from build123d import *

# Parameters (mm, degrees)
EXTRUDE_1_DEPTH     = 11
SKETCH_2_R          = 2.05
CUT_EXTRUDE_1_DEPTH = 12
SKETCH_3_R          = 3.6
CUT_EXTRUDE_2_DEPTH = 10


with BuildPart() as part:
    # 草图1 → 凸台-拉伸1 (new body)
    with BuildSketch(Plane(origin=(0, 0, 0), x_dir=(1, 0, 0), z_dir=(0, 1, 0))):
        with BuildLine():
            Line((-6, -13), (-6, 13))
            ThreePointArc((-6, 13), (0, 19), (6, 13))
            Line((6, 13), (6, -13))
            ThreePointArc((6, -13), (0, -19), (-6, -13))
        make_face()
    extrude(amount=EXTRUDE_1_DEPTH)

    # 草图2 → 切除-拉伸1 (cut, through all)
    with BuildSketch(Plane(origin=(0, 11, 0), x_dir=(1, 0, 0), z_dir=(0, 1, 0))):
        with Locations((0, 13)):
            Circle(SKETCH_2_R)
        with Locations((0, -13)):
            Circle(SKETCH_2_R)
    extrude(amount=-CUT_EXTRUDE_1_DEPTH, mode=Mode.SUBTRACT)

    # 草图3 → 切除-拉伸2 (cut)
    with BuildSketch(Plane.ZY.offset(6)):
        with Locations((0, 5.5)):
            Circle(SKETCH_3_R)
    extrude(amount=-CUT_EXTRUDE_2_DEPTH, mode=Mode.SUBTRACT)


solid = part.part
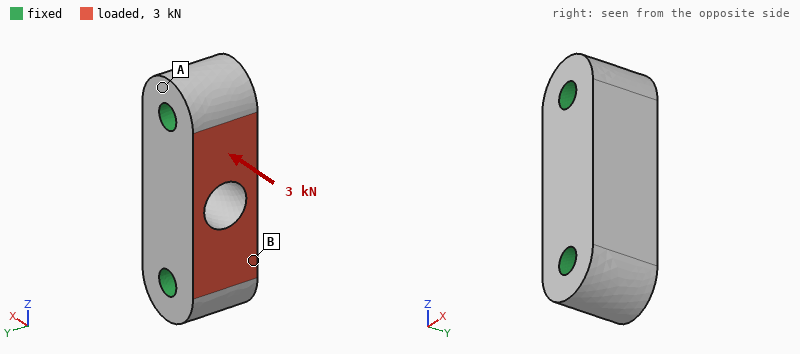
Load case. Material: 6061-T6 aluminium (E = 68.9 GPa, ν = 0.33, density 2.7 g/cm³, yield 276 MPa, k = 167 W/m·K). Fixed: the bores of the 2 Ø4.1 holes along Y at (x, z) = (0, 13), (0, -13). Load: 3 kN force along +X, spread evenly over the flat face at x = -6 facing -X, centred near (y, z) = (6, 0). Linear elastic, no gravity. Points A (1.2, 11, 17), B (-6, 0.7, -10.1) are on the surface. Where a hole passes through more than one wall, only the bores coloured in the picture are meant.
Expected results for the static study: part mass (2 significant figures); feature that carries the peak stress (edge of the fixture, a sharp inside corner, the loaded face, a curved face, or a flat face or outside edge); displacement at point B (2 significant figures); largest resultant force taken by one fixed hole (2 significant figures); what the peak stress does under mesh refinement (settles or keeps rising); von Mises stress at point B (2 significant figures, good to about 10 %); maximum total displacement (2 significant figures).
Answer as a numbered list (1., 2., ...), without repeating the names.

1. 11 g
2. edge of the fixture
3. 3.0 µm
4. 1.5 kN
5. keeps rising
6. 13 MPa
7. 6.5 µm
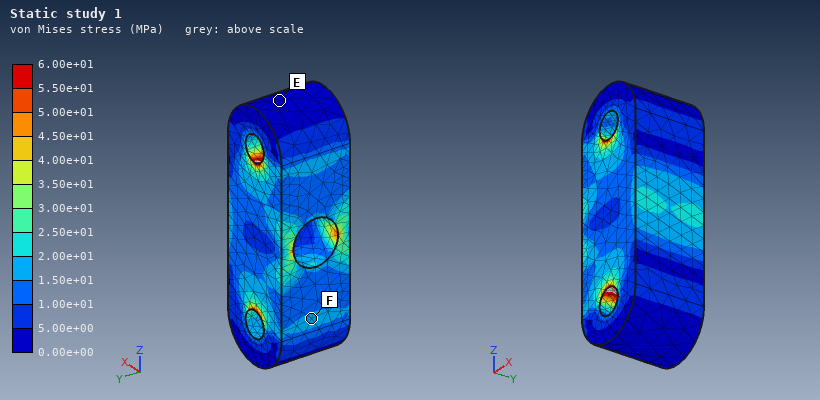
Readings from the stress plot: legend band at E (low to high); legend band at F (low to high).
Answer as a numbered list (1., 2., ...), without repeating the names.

1. 0.00e+00 to 5.00e+00 MPa
2. 1.50e+01 to 2.00e+01 MPa
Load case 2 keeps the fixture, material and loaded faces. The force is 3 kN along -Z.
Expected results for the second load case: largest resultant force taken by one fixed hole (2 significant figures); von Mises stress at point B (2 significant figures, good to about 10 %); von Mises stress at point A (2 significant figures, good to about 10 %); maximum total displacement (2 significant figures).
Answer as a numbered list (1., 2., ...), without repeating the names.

1. 1.6 kN
2. 22 MPa
3. 5.0 MPa
4. 4.1 µm
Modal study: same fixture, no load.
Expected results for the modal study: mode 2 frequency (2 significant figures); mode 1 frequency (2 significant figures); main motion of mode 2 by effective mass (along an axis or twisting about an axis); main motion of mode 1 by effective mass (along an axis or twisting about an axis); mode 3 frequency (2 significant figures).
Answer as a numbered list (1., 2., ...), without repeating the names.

1. 55 kHz
2. 47 kHz
3. along Y
4. along X
5. 60 kHz
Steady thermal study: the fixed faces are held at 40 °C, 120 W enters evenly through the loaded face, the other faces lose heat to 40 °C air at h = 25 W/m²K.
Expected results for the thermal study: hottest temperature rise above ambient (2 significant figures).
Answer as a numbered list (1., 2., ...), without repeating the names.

1. 27 K
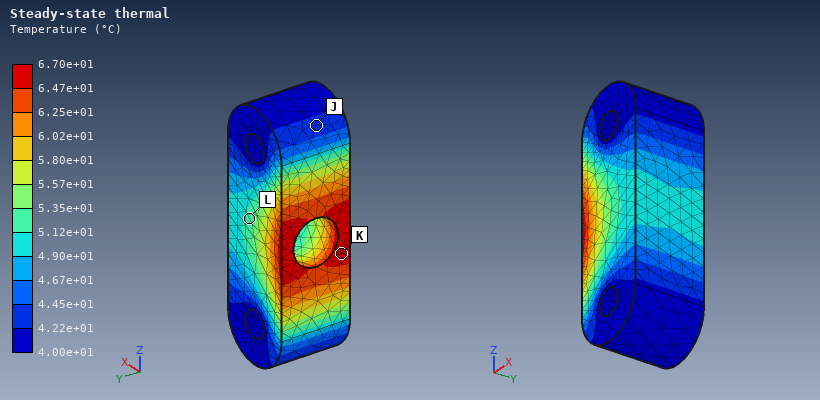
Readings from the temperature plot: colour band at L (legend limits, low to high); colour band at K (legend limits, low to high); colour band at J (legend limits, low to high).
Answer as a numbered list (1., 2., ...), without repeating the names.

1. 5.12e+01 to 5.35e+01 °C
2. 6.47e+01 to 6.70e+01 °C
3. 4.22e+01 to 4.45e+01 °C
